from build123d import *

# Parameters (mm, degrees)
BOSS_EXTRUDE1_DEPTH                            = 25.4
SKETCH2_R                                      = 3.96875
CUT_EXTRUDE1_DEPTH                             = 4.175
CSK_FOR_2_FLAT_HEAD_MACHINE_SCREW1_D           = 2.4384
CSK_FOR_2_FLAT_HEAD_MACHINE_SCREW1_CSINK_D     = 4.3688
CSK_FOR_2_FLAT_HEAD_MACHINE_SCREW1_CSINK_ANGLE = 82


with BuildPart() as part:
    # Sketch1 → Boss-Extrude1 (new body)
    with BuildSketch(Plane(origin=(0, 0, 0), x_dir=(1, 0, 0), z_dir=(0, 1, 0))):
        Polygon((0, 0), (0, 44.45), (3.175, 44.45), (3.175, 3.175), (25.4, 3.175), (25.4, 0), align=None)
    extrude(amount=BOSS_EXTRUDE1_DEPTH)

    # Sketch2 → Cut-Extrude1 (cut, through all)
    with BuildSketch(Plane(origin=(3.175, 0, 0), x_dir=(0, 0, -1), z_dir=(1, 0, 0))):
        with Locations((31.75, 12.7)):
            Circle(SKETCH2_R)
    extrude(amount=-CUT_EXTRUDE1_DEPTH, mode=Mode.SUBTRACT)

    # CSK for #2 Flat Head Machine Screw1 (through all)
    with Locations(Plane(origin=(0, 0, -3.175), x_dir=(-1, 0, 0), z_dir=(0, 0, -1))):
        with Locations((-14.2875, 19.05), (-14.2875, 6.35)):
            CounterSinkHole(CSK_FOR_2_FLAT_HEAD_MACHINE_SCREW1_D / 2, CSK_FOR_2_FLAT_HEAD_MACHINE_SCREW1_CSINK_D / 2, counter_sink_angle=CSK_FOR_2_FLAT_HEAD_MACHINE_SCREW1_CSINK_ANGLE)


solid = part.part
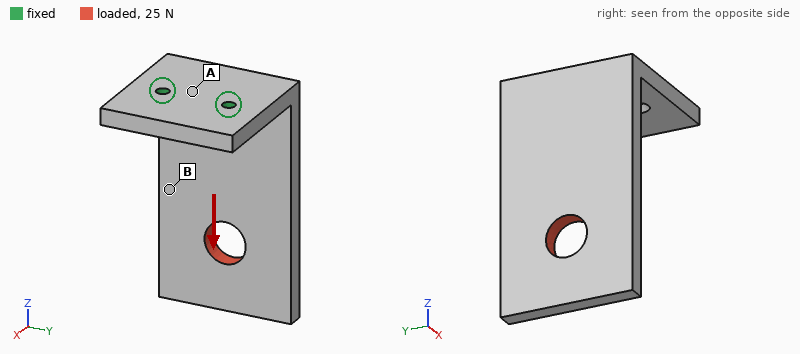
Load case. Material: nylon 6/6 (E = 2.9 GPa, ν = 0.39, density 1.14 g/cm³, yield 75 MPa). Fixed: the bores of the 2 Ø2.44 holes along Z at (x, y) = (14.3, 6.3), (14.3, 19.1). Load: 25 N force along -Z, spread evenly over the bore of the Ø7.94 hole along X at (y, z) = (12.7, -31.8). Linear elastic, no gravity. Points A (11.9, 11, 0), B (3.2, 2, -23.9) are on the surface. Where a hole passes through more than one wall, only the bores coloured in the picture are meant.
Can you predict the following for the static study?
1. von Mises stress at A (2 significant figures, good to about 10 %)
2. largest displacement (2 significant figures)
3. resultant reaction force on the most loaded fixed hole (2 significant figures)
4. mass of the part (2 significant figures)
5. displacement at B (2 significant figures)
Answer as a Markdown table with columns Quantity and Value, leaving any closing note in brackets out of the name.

| Quantity | Value |
|---|---|
| von Mises stress at A | 4.4 MPa |
| largest displacement | 0.58 mm |
| resultant reaction force on the most loaded fixed hole | 13 N |
| mass of the part | 5.9 g |
| displacement at B | 0.31 mm |
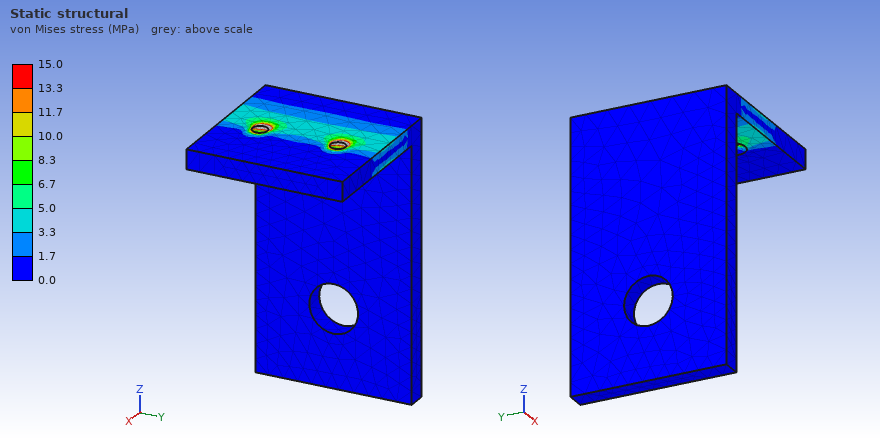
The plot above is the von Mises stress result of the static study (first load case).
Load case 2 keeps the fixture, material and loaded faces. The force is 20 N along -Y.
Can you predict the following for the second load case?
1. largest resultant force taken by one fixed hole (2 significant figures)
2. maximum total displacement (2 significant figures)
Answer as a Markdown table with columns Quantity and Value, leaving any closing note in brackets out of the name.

| Quantity | Value |
|---|---|
| largest resultant force taken by one fixed hole | 45 N |
| maximum total displacement | 0.68 mm |
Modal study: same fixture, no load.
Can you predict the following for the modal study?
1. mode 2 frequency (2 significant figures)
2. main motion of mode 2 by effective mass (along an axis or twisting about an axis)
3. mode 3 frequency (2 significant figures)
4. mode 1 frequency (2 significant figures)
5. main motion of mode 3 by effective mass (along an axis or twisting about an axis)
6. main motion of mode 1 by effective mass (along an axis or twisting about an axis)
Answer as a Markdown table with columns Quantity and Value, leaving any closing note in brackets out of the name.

| Quantity | Value |
|---|---|
| mode 2 frequency | 640 Hz |
| main motion of mode 2 by effective mass | along Y |
| mode 3 frequency | 1400 Hz |
| mode 1 frequency | 310 Hz |
| main motion of mode 3 by effective mass | along Z |
| main motion of mode 1 by effective mass | along X |
